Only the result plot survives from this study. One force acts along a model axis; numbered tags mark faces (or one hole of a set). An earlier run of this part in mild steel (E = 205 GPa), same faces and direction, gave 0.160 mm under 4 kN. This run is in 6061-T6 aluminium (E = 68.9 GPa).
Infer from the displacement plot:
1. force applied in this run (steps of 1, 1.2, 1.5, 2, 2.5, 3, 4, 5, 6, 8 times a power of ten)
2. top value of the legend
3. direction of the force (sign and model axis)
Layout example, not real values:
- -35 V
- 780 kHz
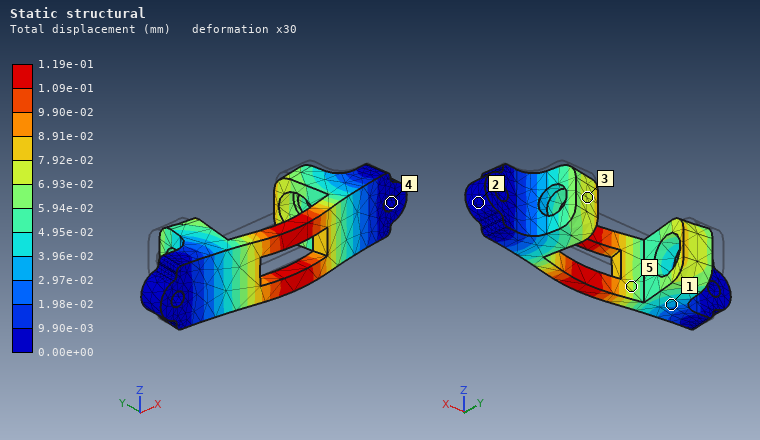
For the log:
- 1 kN
- 1.19e-01 mm
- -Y
